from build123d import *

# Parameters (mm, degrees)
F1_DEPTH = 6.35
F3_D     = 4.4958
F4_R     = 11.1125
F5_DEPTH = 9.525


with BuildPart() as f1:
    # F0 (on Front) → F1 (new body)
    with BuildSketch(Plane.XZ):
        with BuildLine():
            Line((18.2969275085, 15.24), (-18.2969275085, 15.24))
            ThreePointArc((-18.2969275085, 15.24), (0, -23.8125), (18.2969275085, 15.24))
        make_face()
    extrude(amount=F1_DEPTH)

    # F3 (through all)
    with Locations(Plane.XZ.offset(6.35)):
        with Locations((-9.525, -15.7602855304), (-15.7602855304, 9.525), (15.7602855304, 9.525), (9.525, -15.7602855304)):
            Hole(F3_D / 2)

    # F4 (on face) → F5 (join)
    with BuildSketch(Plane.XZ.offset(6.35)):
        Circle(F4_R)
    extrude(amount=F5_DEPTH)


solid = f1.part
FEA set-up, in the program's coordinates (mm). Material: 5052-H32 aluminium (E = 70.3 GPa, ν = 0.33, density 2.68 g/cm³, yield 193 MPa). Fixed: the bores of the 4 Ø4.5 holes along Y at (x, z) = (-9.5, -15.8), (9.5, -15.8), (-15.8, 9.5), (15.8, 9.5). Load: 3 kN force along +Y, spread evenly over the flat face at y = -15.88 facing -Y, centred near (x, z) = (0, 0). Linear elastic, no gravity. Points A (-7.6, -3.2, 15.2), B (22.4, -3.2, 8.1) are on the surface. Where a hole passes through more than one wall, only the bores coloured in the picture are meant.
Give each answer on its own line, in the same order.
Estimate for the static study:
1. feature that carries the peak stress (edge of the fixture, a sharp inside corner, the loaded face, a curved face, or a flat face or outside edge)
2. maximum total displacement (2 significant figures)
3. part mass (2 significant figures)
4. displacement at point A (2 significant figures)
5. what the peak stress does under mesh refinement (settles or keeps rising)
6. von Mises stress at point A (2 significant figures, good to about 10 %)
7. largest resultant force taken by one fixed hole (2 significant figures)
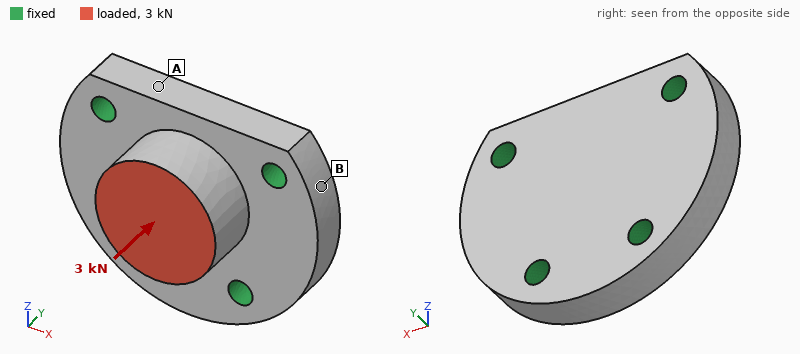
edge of the fixture
8.3 µm
35 g
4.1 µm
keeps rising
13 MPa
920 N
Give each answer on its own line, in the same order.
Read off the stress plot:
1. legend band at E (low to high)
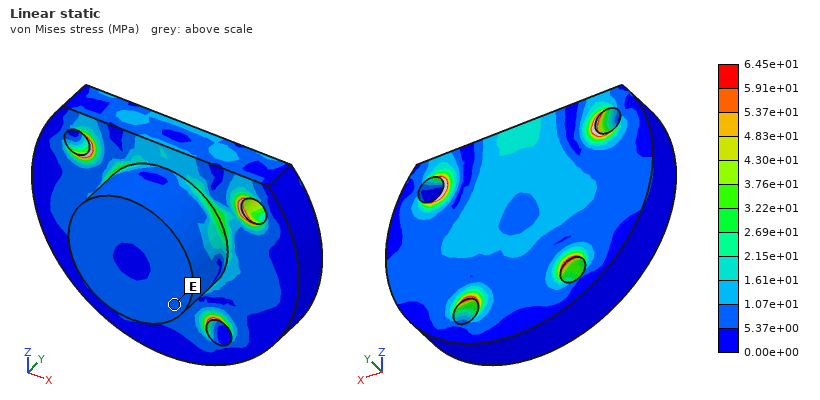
5.37e+00 to 1.07e+01 MPa
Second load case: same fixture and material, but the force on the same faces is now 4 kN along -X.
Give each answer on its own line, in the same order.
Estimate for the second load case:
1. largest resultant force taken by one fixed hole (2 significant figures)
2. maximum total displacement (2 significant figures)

1.8 kN
20 µm
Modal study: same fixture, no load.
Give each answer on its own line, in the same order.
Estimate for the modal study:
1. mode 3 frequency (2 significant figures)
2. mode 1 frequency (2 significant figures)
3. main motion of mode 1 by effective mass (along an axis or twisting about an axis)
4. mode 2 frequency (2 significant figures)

30 kHz
24 kHz
along Y
28 kHz
